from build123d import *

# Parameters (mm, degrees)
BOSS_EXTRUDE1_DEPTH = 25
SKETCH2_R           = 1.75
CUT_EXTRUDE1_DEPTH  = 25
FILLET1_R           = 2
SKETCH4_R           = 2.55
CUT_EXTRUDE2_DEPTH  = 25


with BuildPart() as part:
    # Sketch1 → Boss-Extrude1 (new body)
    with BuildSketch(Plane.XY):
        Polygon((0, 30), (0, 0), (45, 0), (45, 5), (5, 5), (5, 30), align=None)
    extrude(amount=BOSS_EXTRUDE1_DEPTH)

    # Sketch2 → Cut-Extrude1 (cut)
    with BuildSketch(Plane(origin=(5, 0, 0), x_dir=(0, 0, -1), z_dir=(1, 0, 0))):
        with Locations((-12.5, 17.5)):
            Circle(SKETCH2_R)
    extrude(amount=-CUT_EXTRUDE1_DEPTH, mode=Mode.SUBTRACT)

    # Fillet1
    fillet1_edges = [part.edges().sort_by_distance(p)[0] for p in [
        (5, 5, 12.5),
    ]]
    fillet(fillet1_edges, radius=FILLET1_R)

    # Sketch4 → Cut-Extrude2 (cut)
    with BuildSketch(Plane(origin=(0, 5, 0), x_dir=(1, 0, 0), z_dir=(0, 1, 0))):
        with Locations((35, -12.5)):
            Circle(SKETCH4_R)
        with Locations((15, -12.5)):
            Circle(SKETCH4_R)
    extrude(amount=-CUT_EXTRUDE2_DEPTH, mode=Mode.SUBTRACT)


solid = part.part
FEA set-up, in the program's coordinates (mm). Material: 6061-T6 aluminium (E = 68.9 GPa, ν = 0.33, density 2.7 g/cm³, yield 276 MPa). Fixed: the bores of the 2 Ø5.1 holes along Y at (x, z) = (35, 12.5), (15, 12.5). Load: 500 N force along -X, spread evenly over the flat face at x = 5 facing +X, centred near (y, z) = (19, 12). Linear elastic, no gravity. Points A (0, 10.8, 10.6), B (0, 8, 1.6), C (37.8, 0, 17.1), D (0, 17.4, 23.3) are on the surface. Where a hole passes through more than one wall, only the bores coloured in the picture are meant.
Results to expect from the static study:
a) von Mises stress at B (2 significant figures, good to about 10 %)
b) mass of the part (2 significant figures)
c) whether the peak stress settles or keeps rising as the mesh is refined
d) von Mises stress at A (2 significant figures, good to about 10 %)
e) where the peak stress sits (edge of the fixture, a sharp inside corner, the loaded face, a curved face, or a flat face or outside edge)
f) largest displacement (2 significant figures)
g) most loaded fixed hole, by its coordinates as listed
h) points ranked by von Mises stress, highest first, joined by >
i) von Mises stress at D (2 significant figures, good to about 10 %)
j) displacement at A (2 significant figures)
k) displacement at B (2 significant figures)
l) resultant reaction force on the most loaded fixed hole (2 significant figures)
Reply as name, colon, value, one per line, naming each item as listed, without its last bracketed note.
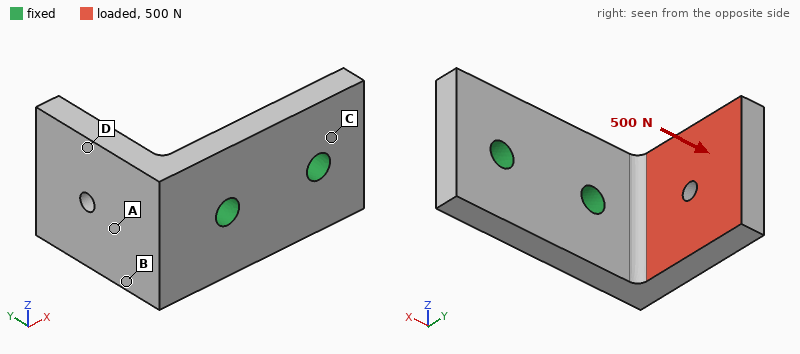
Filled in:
von Mises stress at B: 50 MPa
mass of the part: 23 g
whether the peak stress settles or keeps rising as the mesh is refined: keeps rising
von Mises stress at A: 33 MPa
where the peak stress sits: edge of the fixture
largest displacement: 0.20 mm
most loaded fixed hole, by its coordinates as listed: (15, 12.5)
points ranked by von Mises stress, highest first, joined by >: B > A > D > C
von Mises stress at D: 18 MPa
displacement at A: 0.069 mm
displacement at B: 0.056 mm
resultant reaction force on the most loaded fixed hole: 440 N
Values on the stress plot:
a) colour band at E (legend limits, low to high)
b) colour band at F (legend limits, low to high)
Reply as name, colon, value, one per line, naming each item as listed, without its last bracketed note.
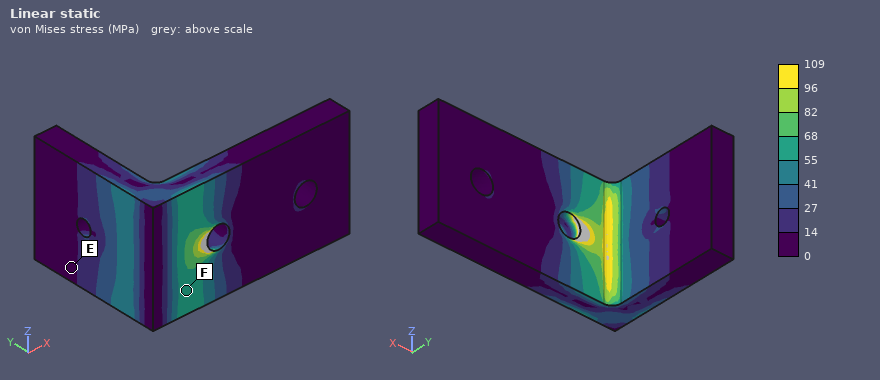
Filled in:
colour band at E: 0 to 14 MPa
colour band at F: 55 to 68 MPa
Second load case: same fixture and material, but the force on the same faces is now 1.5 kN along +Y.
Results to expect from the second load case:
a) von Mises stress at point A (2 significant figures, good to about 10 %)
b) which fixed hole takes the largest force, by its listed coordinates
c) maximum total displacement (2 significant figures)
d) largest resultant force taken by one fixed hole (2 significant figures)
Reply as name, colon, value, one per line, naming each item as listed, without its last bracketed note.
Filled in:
von Mises stress at point A: 16 MPa
which fixed hole takes the largest force, by its listed coordinates: (15, 12.5)
maximum total displacement: 79 µm
largest resultant force taken by one fixed hole: 1.7 kN
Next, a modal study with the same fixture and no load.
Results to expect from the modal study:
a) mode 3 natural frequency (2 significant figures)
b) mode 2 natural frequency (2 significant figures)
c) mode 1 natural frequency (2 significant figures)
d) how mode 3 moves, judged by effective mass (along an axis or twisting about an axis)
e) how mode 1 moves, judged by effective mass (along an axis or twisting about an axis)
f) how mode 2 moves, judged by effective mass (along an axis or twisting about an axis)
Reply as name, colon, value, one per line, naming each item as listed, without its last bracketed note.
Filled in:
mode 3 natural frequency: 11 kHz
mode 2 natural frequency: 4700 Hz
mode 1 natural frequency: 3400 Hz
how mode 3 moves, judged by effective mass: along Y
how mode 1 moves, judged by effective mass: along X
how mode 2 moves, judged by effective mass: along Z
